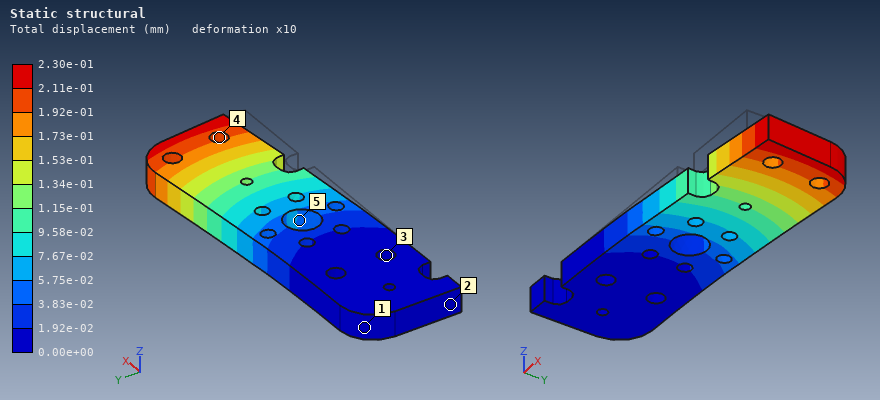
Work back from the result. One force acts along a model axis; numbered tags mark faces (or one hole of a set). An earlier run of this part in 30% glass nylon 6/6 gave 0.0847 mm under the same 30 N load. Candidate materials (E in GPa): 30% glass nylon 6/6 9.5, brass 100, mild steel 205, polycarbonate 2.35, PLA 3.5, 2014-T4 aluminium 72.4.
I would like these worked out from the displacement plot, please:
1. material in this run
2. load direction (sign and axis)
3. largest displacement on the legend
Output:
PLA
+Y
2.30e-01 mm
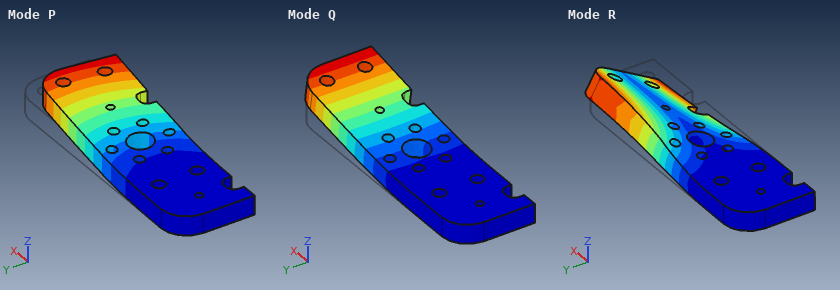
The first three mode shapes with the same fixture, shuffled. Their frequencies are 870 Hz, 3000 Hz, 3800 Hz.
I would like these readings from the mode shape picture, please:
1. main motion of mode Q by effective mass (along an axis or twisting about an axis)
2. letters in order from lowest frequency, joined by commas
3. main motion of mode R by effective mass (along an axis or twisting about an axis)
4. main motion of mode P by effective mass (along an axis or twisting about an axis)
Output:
along Z
Q, P, R
twisting about X
along Y
